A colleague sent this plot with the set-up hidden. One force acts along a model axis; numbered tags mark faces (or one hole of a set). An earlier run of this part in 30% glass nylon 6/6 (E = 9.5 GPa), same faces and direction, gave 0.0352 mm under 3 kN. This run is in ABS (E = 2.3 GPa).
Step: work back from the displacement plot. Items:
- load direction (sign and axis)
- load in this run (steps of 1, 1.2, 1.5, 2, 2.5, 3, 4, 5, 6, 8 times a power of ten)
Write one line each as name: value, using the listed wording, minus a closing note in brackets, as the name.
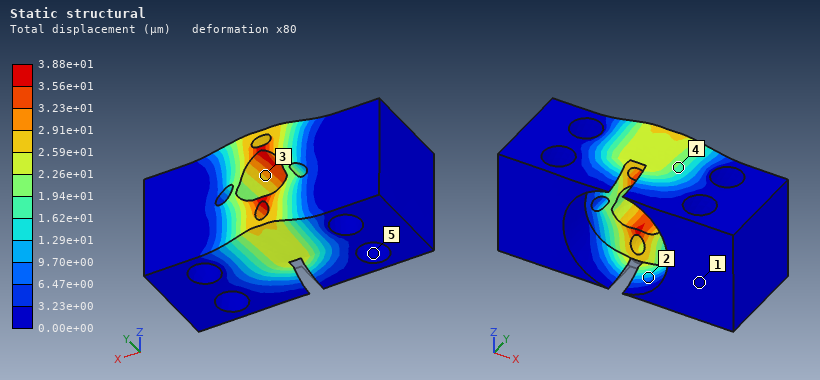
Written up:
load direction: +Z
load in this run: 800 N
